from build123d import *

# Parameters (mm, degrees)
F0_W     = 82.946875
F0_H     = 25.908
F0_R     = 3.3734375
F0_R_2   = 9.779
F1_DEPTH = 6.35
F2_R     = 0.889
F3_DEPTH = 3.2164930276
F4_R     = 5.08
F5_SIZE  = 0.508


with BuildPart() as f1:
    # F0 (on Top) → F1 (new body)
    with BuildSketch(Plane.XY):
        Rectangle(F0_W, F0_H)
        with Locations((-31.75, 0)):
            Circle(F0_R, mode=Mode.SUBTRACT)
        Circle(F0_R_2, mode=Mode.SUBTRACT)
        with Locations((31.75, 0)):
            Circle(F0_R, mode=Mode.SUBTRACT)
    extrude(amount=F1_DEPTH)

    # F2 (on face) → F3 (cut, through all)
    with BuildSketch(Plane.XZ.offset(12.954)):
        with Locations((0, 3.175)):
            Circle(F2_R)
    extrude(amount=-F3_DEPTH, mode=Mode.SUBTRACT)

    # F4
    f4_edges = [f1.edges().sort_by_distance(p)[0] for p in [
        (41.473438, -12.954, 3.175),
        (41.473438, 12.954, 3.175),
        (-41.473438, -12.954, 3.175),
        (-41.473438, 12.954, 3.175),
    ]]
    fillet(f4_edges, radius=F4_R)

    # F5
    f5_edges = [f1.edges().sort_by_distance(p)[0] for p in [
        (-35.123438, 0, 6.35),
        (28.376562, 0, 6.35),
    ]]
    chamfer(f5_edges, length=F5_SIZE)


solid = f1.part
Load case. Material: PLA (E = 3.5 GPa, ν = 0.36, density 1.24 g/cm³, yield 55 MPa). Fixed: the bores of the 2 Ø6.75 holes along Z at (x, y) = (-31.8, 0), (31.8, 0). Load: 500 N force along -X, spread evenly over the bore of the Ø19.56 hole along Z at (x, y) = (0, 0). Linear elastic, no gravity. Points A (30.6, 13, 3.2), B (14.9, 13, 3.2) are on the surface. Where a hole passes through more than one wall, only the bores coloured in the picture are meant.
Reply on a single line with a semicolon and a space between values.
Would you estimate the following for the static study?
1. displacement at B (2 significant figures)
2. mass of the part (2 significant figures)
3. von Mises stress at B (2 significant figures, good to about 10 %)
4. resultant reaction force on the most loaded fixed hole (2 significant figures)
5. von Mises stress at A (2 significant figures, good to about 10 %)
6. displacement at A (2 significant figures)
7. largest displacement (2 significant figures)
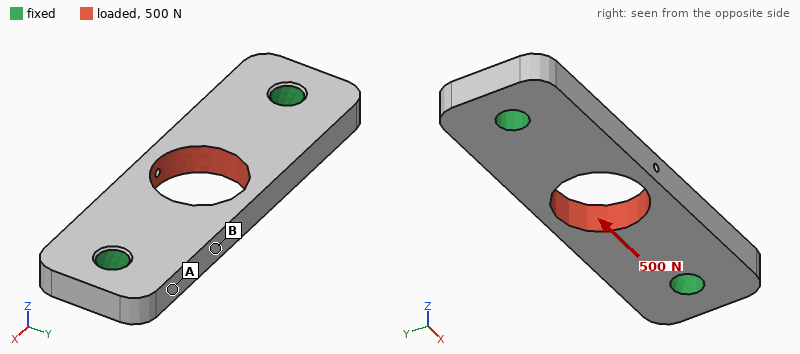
11 µm; 14 g; 1.5 MPa; 250 N; 0.51 MPa; 5.8 µm; 17 µm
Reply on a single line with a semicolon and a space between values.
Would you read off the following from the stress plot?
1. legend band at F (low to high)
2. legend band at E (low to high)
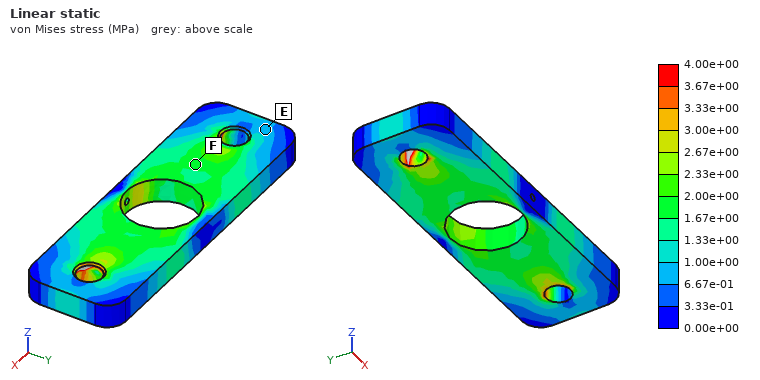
1.67e+00 to 2.00e+00 MPa; 6.67e-01 to 1.00e+00 MPa
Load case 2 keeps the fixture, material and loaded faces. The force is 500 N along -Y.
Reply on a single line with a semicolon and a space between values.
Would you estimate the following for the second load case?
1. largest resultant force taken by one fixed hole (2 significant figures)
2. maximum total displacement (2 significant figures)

250 N; 93 µm
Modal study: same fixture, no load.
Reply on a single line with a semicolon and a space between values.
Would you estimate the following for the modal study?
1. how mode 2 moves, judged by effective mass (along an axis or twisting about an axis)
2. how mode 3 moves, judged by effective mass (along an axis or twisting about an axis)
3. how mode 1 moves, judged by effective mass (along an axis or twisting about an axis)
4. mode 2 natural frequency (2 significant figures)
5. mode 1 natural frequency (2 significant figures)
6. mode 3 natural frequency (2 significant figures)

twisting about X; along Y; along Z; 4000 Hz; 2900 Hz; 5900 Hz
